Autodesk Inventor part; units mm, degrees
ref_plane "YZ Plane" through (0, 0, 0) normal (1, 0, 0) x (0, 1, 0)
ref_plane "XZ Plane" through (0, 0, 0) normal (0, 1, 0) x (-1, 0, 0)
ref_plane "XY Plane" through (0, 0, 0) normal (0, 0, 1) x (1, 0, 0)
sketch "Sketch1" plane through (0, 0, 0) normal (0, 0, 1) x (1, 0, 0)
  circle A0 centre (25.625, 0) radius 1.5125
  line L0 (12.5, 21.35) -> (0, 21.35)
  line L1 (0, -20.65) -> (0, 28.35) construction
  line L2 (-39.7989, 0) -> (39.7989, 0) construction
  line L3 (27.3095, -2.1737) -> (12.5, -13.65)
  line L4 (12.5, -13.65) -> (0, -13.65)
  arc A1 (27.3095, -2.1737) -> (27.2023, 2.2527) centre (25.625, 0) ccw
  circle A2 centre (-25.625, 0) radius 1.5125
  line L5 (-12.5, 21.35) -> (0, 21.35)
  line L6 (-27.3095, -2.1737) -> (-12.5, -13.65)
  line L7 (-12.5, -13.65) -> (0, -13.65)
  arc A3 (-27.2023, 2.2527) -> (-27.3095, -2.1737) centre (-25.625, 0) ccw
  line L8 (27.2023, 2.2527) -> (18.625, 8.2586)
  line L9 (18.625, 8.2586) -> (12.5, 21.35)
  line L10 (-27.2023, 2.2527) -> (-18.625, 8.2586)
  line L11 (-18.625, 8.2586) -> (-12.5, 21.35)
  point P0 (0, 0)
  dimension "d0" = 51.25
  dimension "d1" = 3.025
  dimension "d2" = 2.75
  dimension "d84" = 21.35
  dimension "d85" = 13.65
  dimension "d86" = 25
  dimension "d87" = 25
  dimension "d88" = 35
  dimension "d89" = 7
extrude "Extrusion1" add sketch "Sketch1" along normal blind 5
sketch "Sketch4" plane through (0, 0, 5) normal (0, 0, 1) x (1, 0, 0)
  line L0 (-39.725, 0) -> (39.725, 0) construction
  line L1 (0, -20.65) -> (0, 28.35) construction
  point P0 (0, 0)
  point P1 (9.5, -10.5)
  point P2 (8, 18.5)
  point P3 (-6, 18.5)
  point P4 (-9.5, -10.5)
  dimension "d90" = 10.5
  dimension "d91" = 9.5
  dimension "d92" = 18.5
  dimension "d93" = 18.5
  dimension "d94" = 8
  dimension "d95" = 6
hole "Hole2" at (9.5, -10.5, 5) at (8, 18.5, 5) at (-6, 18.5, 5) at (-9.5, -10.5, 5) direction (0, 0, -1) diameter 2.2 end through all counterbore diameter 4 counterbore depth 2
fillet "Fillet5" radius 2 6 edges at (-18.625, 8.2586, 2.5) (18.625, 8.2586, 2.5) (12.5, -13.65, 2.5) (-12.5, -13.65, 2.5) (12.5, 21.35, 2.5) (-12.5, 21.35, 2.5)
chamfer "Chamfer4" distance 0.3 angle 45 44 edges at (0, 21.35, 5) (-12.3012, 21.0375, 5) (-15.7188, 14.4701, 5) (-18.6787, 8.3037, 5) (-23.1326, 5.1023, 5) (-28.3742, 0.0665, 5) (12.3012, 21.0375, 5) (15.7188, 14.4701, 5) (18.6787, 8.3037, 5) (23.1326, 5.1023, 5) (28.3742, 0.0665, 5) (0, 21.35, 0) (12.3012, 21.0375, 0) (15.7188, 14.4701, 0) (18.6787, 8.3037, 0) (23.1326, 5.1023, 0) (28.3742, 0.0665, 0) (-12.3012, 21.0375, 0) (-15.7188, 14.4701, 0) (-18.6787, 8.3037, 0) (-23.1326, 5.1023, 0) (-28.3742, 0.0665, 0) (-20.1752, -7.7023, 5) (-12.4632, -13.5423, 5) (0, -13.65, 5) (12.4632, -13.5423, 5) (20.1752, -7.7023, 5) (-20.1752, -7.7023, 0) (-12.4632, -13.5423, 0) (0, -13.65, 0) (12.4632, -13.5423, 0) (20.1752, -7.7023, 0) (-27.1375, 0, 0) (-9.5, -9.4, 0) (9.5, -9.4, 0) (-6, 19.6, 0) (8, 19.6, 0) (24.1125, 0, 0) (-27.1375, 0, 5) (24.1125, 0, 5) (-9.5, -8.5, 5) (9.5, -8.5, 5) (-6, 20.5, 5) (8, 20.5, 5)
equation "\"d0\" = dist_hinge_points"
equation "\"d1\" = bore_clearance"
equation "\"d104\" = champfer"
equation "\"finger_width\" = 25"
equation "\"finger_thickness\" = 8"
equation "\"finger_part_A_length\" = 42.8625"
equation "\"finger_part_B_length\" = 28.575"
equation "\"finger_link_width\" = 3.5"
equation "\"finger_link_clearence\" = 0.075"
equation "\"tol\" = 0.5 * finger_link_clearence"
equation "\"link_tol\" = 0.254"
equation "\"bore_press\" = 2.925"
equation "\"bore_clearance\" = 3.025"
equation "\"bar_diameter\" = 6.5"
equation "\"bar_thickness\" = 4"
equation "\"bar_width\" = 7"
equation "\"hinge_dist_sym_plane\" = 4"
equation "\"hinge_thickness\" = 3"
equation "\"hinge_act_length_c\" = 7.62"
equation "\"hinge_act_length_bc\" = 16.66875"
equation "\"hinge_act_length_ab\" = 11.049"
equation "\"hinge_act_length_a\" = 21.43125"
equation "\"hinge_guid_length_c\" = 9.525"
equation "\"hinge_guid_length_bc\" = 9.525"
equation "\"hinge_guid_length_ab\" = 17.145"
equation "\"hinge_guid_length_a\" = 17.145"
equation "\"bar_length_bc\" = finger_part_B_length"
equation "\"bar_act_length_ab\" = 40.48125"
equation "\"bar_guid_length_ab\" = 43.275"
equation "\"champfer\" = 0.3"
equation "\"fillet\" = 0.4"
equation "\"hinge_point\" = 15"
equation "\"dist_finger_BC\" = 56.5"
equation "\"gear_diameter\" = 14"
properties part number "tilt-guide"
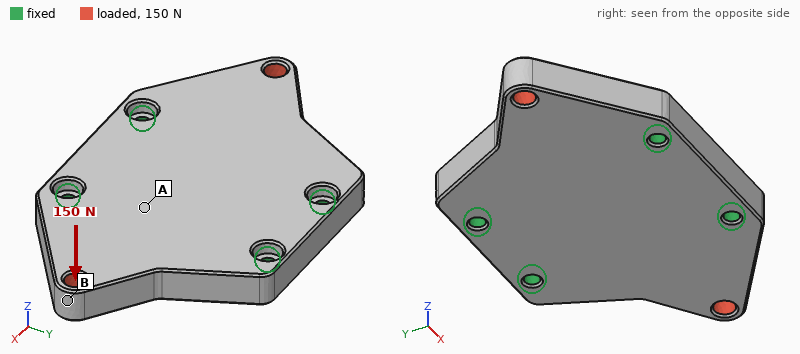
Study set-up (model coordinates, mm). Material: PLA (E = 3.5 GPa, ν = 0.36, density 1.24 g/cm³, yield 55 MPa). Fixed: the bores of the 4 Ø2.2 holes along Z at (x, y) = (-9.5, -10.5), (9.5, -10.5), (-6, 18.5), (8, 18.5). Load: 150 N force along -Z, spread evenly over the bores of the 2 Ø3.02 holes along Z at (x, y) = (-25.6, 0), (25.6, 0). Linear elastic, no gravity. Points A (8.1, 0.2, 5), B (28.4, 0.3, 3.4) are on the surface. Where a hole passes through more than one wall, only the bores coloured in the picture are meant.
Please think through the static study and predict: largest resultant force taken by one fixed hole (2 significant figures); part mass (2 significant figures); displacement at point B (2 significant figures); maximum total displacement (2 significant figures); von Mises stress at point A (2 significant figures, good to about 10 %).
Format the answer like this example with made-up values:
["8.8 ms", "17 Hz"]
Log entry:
["86 N", "8.3 g", "0.37 mm", "0.39 mm", "8.8 MPa"]
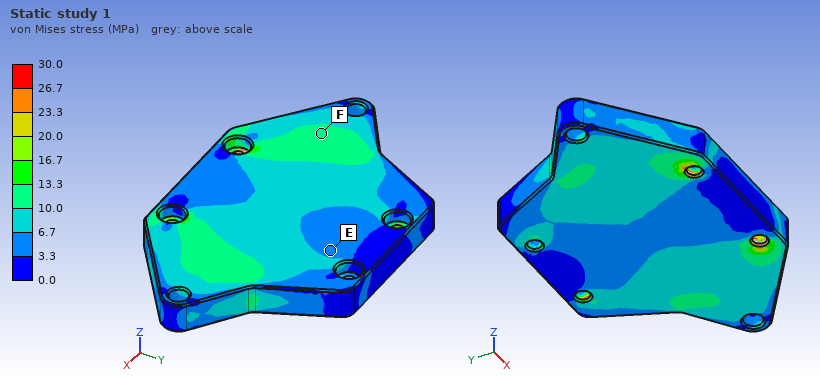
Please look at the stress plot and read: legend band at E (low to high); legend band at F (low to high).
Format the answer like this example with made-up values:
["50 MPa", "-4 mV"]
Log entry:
["3.3 to 6.7 MPa", "10.0 to 13.3 MPa"]
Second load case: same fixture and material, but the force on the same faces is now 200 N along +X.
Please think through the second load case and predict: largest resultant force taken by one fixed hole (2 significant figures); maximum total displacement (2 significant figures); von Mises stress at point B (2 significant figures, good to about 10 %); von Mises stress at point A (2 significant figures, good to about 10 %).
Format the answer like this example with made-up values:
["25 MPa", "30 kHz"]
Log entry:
["63 N", "19 µm", "4.0 MPa", "0.70 MPa"]
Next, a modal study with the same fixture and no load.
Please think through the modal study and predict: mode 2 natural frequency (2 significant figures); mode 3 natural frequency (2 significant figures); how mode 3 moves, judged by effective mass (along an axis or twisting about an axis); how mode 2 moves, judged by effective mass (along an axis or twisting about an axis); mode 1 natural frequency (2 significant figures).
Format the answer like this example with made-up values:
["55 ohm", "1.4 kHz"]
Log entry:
["3600 Hz", "7000 Hz", "along Z", "along Z", "3400 Hz"]
